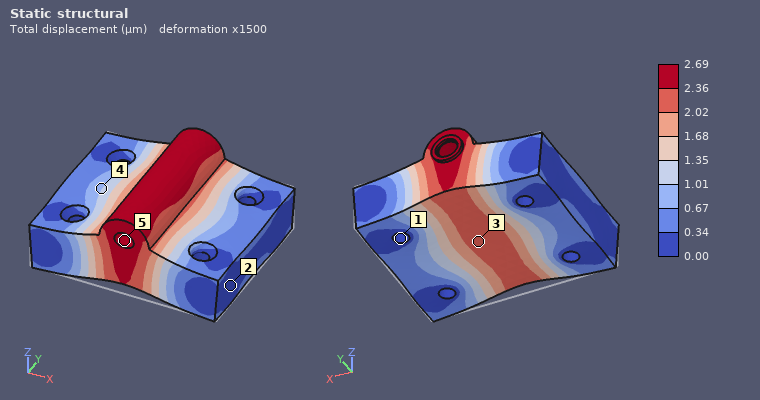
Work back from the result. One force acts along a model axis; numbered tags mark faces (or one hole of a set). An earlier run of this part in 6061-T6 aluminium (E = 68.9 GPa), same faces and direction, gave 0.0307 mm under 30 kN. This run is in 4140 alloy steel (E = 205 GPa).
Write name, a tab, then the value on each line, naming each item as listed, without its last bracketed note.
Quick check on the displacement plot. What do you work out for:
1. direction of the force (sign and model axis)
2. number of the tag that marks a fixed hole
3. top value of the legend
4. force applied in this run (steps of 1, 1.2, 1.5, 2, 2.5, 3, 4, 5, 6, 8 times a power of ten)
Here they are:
direction of the force	+Z
number of the tag that marks a fixed hole	1
top value of the legend	2.69 µm
force applied in this run	8 kN
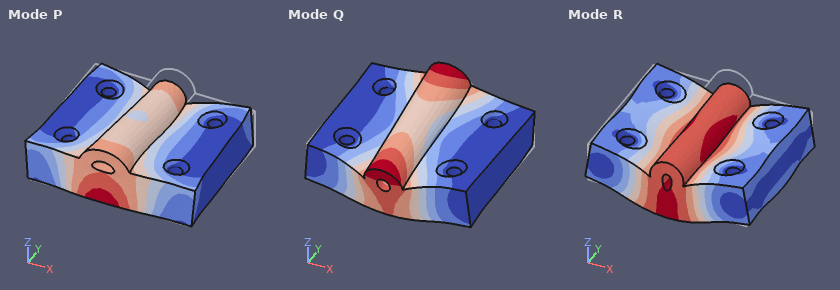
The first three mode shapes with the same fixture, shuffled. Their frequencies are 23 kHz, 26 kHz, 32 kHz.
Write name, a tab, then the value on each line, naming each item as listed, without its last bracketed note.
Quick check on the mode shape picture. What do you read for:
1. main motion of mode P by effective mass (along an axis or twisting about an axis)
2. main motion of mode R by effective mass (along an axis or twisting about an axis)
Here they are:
main motion of mode P by effective mass	along Y
main motion of mode R by effective mass	along Z
